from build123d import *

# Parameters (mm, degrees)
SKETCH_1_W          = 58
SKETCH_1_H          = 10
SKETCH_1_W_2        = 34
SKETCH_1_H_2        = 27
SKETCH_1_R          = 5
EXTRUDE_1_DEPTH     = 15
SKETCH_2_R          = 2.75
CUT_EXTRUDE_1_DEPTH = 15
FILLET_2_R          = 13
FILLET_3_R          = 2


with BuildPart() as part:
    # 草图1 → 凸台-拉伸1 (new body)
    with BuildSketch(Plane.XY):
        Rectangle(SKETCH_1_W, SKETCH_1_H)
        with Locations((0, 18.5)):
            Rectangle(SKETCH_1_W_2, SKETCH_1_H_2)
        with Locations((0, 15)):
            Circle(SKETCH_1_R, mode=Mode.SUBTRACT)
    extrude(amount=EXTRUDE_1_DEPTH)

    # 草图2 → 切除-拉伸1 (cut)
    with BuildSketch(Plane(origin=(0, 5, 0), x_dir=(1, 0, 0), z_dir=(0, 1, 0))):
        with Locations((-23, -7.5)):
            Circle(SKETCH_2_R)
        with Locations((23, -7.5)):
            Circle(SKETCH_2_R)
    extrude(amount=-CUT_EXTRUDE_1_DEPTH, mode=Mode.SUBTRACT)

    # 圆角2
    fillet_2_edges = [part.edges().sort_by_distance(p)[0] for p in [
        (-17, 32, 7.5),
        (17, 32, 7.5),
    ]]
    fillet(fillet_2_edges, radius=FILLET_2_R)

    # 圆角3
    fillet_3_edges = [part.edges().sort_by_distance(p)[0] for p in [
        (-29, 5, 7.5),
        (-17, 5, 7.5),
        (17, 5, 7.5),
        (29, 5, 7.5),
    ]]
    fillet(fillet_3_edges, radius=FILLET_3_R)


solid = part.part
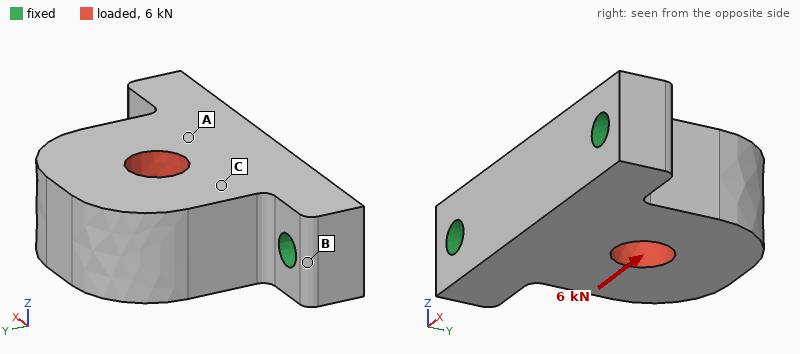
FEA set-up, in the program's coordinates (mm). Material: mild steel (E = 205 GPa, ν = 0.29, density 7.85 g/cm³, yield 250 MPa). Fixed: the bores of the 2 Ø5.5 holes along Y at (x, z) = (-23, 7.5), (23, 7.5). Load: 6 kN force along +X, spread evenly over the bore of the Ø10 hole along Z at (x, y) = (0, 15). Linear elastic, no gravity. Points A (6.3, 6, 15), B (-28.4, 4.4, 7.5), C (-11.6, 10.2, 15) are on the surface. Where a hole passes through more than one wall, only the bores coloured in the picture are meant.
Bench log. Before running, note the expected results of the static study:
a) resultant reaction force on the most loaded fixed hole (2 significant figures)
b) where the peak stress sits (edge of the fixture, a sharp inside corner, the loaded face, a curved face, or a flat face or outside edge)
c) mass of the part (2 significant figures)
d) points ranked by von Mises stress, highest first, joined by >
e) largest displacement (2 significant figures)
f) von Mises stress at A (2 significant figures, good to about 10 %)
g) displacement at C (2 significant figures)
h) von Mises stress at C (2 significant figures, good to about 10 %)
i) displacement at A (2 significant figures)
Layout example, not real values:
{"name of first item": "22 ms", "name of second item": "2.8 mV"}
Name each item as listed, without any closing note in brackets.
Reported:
{"resultant reaction force on the most loaded fixed hole": "3.7 kN", "where the peak stress sits": "a curved face", "mass of the part": "150 g", "points ranked by von Mises stress, highest first, joined by >": "C > A > B", "largest displacement": "6.9 µm", "von Mises stress at A": "18 MPa", "displacement at C": "2.9 µm", "von Mises stress at C": "26 MPa", "displacement at A": "1.8 µm"}
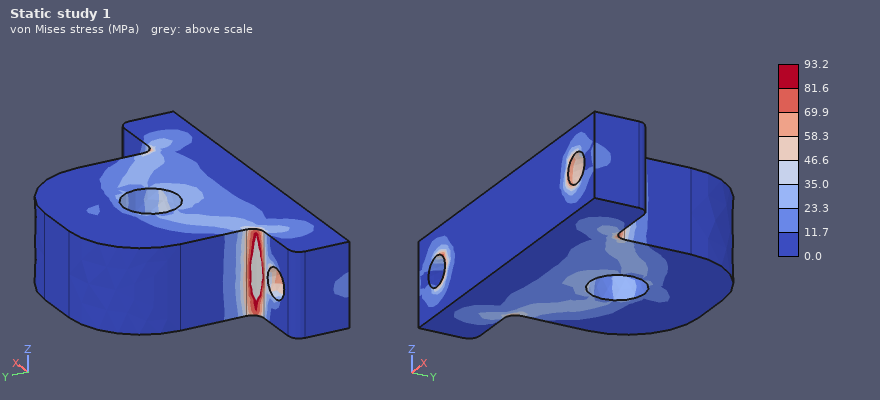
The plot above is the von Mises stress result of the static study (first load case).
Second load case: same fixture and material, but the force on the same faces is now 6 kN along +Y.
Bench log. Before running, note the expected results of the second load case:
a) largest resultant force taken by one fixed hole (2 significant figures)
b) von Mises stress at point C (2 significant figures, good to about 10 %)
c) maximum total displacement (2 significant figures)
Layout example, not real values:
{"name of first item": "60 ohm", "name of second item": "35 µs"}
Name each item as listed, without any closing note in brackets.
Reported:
{"largest resultant force taken by one fixed hole": "3.3 kN", "von Mises stress at point C": "18 MPa", "maximum total displacement": "4.9 µm"}
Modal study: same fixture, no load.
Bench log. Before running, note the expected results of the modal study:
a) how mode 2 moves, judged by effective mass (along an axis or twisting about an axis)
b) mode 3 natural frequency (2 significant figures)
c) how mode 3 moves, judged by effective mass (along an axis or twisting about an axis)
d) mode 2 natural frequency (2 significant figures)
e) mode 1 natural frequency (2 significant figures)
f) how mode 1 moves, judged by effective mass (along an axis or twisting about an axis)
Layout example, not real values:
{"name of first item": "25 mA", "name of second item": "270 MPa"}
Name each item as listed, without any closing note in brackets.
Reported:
{"how mode 2 moves, judged by effective mass": "along X", "mode 3 natural frequency": "17 kHz", "how mode 3 moves, judged by effective mass": "along Y", "mode 2 natural frequency": "15 kHz", "mode 1 natural frequency": "5800 Hz", "how mode 1 moves, judged by effective mass": "along Z"}
